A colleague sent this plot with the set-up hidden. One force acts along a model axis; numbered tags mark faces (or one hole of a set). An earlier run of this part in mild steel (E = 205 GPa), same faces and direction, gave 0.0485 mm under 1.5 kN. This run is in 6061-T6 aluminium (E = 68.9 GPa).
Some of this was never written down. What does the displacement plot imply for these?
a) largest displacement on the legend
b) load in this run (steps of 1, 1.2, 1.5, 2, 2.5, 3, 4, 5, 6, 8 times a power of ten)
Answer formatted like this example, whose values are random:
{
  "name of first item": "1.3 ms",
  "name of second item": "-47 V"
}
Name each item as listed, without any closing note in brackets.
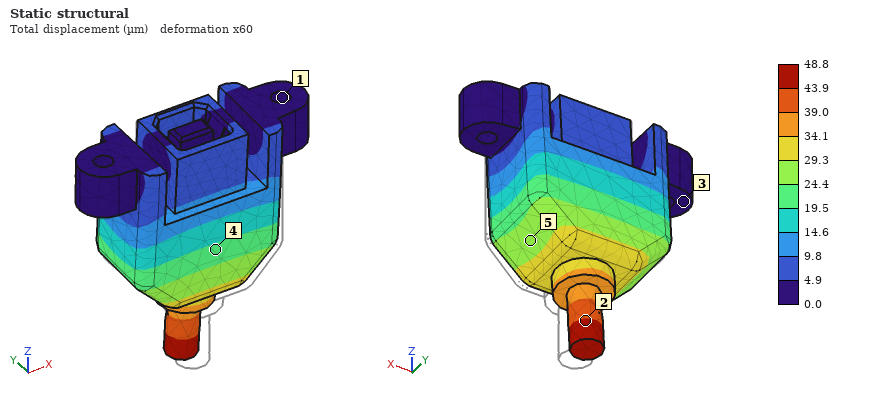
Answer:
{
  "largest displacement on the legend": "48.8 µm",
  "load in this run": "500 N"
}
